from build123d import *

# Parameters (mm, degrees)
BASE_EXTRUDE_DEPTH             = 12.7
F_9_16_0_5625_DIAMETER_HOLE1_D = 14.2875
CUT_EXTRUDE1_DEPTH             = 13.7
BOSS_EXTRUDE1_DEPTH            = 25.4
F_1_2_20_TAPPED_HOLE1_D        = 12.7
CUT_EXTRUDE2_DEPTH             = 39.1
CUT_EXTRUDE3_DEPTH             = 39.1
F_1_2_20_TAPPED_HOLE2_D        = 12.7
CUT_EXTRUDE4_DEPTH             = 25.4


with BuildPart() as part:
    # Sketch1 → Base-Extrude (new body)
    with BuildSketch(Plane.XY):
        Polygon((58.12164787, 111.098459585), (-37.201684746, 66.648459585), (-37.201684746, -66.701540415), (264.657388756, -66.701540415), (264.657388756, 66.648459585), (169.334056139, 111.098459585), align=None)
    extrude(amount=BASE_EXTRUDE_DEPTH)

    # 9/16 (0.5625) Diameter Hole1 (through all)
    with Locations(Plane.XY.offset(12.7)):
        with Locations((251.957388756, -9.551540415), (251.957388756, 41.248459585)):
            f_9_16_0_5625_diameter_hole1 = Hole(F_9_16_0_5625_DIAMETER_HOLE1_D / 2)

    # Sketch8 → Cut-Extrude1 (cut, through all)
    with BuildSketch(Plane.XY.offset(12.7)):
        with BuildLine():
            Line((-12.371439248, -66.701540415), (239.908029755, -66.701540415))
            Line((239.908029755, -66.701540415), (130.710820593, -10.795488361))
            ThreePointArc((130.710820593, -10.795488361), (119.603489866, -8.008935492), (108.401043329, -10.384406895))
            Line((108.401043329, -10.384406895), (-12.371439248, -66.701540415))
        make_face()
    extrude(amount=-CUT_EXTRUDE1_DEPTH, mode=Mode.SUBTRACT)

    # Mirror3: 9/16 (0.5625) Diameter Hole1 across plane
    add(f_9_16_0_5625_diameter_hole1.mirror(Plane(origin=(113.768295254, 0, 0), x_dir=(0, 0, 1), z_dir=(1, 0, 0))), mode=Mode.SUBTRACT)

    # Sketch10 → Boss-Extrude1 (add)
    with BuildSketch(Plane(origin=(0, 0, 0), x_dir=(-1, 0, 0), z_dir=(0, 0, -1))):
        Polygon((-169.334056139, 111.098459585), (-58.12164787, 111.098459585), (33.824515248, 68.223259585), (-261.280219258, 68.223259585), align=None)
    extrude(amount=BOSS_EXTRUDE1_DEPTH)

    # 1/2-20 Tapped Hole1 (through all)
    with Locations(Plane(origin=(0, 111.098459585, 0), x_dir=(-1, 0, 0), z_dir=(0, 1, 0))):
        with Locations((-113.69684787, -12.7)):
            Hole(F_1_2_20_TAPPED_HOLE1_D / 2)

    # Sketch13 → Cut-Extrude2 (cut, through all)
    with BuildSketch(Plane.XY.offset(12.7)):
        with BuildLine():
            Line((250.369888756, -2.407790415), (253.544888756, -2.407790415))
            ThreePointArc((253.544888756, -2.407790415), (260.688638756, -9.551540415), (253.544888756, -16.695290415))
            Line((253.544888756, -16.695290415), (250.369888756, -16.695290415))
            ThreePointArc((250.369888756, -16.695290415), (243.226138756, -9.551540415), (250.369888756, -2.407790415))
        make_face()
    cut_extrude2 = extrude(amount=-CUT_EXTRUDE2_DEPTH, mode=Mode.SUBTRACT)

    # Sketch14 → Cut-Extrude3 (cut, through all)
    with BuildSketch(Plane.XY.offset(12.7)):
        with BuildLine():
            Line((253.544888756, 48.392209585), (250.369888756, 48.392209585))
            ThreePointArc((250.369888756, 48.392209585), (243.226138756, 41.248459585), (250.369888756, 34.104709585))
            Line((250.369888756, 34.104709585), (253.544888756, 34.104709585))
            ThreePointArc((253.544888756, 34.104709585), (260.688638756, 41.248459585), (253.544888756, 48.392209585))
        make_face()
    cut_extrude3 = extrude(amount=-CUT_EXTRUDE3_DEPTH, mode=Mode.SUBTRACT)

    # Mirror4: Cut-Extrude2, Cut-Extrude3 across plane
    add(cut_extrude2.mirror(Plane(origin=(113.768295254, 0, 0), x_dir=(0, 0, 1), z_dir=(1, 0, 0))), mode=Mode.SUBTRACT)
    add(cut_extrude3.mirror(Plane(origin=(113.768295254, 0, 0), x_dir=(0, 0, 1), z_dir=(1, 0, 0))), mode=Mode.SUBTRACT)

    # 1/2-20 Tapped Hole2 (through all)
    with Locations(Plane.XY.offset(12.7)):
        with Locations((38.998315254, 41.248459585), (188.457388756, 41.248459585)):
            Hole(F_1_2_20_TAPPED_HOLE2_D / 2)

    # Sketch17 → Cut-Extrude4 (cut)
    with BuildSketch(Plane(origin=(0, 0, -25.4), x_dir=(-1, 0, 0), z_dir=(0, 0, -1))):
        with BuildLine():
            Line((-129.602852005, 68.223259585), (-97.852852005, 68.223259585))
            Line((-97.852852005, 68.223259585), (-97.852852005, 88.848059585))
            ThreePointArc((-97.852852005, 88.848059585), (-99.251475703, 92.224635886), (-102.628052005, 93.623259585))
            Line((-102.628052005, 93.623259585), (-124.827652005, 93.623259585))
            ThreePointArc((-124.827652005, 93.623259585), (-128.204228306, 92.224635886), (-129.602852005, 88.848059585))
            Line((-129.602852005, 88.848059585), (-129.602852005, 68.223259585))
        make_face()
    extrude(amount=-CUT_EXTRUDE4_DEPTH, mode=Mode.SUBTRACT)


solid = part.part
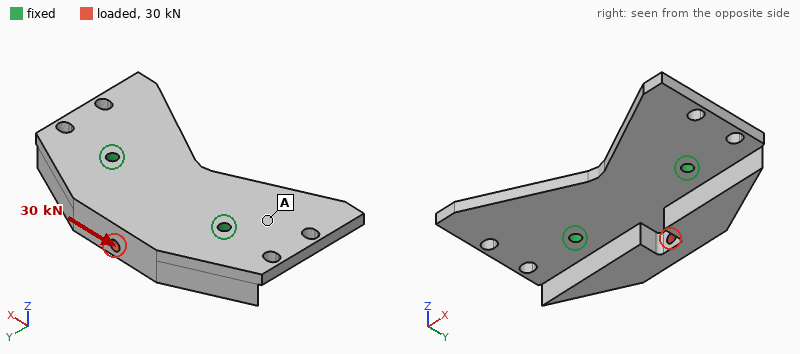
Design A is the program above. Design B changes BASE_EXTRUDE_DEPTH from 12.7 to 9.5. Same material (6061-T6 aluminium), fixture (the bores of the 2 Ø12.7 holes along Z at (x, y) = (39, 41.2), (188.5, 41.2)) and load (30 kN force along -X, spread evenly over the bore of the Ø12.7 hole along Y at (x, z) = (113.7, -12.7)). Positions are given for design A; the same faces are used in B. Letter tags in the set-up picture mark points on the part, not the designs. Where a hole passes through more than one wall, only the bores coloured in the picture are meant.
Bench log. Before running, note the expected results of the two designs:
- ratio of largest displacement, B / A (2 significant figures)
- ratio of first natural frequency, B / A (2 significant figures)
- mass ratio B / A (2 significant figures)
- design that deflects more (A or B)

1.5
0.77
0.82
B
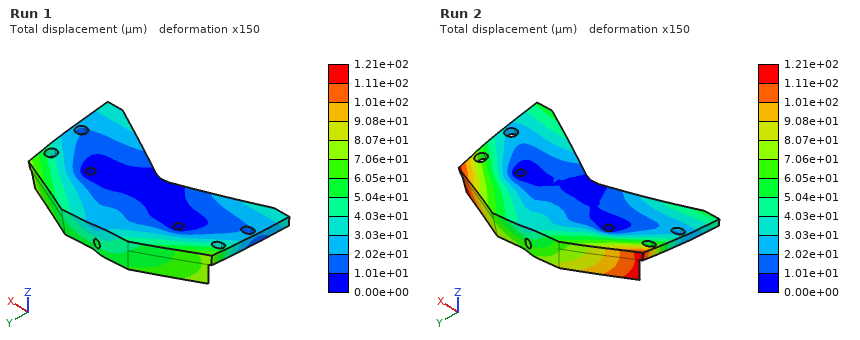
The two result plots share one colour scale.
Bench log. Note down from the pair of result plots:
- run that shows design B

Run 2
